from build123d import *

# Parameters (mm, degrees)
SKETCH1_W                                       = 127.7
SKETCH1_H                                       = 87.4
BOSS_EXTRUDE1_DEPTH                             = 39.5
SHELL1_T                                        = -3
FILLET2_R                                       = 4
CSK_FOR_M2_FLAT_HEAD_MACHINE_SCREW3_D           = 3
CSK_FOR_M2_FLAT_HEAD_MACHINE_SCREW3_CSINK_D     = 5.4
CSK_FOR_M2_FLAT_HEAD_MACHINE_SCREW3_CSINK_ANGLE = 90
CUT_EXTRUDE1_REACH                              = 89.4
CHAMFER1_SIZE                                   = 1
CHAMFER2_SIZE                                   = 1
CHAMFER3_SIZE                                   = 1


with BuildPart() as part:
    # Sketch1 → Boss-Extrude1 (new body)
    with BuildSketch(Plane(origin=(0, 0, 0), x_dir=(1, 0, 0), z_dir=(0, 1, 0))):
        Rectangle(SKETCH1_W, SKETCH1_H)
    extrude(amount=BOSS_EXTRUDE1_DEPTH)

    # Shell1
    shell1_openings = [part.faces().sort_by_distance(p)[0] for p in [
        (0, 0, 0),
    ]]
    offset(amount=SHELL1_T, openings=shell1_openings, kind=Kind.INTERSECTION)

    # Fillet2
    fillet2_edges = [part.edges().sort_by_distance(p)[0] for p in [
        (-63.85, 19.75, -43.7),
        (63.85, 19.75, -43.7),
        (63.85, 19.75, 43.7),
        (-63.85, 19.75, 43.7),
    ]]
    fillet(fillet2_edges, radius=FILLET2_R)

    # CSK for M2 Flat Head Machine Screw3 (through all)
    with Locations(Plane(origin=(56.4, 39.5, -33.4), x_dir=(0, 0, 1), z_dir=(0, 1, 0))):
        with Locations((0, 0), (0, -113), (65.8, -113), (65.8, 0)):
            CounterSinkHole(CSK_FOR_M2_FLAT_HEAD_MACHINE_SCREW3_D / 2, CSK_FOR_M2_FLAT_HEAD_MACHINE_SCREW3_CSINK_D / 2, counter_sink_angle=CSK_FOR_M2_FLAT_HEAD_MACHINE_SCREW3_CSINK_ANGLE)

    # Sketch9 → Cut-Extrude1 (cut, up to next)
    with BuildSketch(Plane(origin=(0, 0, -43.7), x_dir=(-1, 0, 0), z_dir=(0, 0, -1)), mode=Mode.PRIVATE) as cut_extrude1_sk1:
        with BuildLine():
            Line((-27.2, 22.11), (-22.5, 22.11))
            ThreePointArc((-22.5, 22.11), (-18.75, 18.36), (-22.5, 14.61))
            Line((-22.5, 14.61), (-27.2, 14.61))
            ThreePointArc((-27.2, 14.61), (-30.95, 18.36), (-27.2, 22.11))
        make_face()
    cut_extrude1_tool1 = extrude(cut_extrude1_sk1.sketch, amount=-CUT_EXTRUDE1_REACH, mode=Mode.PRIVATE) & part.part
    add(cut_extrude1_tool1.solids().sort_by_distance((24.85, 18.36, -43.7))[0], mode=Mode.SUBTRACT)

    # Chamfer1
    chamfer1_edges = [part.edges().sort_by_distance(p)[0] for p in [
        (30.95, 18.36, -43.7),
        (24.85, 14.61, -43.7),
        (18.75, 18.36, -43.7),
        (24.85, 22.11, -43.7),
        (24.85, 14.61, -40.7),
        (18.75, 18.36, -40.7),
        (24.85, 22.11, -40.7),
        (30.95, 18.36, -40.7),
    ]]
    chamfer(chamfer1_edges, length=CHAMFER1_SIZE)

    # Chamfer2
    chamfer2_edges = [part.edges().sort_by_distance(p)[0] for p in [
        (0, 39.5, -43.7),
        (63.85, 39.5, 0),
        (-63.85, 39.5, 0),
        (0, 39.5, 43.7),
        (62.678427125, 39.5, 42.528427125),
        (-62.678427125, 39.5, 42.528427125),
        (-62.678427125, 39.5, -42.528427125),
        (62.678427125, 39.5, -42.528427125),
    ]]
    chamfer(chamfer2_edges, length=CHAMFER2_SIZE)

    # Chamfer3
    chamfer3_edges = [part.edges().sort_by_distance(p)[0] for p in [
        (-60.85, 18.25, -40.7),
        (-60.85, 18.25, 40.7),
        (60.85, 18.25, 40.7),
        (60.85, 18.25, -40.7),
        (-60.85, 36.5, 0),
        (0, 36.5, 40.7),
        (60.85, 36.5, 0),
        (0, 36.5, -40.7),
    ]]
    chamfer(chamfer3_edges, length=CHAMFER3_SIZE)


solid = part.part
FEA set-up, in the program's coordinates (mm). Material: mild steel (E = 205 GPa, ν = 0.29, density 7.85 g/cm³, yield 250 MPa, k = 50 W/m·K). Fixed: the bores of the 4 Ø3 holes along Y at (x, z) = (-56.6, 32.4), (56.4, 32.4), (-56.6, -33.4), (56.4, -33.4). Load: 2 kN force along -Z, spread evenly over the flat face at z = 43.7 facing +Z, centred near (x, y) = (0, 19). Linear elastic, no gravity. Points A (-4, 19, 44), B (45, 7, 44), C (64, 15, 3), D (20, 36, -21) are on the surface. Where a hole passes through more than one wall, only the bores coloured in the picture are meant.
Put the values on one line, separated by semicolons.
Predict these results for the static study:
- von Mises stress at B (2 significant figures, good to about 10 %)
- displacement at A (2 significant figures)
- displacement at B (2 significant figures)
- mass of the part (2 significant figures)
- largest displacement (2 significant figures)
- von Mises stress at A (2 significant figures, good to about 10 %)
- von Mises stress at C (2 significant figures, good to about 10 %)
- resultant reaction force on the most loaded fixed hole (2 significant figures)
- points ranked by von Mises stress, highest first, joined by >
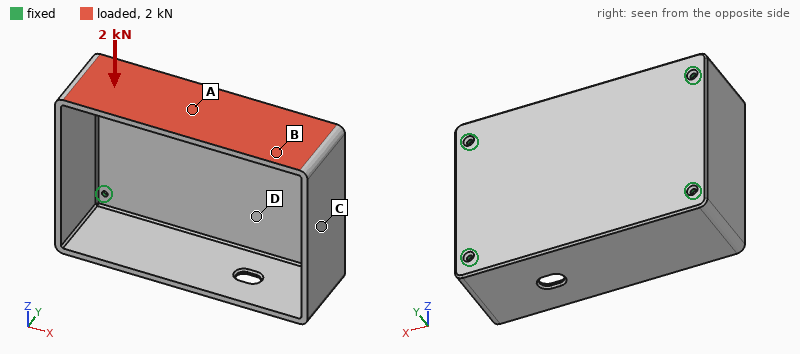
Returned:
77 MPa; 0.13 mm; 0.088 mm; 620 g; 0.28 mm; 29 MPa; 15 MPa; 650 N; B > A > C > D
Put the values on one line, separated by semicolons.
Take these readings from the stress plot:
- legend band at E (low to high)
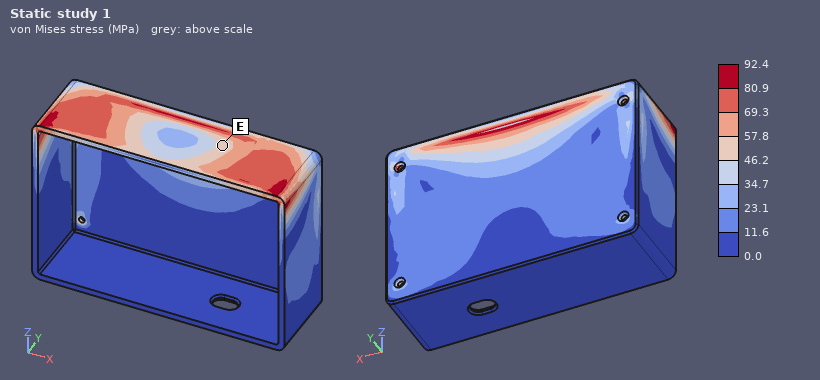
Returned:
46.2 to 57.8 MPa
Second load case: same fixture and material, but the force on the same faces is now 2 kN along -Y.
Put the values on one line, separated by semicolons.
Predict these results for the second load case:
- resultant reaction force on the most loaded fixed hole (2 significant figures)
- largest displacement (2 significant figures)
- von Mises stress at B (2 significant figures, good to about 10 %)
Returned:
1.3 kN; 46 µm; 17 MPa
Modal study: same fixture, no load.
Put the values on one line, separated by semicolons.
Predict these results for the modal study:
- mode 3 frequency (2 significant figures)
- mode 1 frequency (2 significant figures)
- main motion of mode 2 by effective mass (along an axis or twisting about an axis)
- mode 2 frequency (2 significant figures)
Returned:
2300 Hz; 1500 Hz; along Z; 1800 Hz
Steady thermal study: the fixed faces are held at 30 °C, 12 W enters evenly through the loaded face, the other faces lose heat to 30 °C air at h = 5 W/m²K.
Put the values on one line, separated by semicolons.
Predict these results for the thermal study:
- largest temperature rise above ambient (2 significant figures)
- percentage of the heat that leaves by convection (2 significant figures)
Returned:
27 K; 17 %
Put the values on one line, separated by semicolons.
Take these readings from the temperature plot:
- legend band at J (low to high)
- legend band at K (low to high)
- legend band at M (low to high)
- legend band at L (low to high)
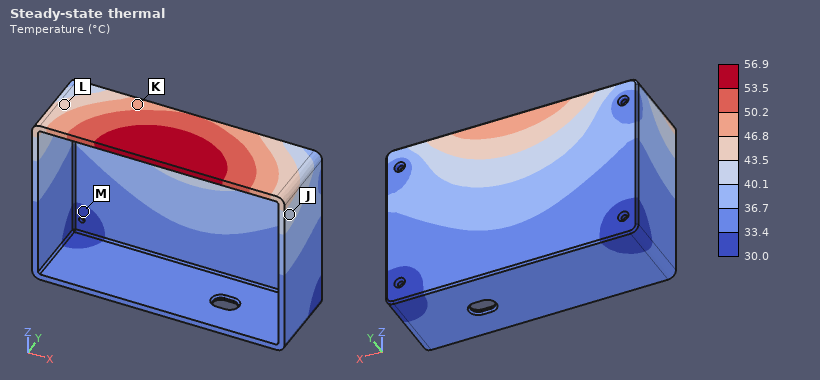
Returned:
40.1 to 43.5 °C; 46.8 to 50.2 °C; 30.0 to 33.4 °C; 43.5 to 46.8 °C
